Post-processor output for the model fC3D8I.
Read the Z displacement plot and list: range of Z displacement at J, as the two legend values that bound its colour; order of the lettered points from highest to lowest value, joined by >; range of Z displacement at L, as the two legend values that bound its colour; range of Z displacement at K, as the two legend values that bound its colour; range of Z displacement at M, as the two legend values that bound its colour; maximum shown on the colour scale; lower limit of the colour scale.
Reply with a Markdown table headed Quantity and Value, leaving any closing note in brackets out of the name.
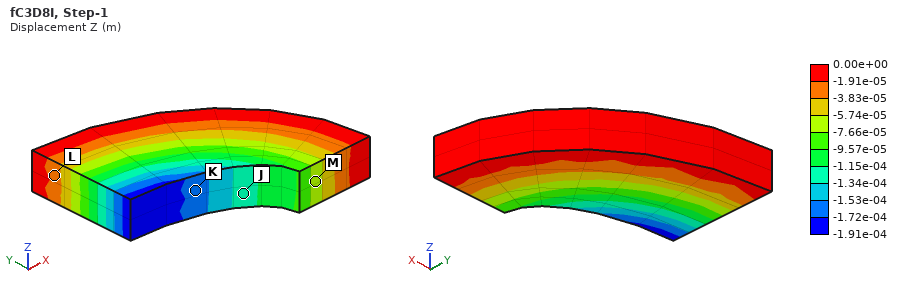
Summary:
| Quantity | Value |
|---|---|
| range of Z displacement at J, as the two legend values that bound its colour | -1.34e-04 to -1.15e-04 m |
| order of the lettered points from highest to lowest value, joined by > | L > M > J > K |
| range of Z displacement at L, as the two legend values that bound its colour | -3.83e-05 to -1.91e-05 m |
| range of Z displacement at K, as the two legend values that bound its colour | -1.72e-04 to -1.53e-04 m |
| range of Z displacement at M, as the two legend values that bound its colour | -7.66e-05 to -5.74e-05 m |
| maximum shown on the colour scale | 0.00e+00 m |
| lower limit of the colour scale | -1.91e-04 m |
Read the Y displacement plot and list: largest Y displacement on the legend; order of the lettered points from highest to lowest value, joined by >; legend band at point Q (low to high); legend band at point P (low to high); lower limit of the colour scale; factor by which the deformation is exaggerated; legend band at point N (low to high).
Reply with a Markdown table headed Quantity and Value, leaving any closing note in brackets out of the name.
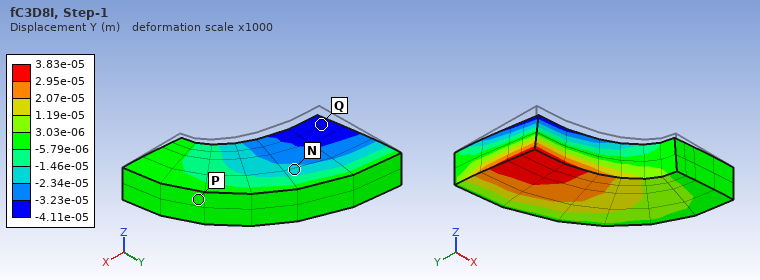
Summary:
| Quantity | Value |
|---|---|
| largest Y displacement on the legend | 3.83e-05 m |
| order of the lettered points from highest to lowest value, joined by > | P > N > Q |
| legend band at point Q | -4.11e-05 to -3.23e-05 m |
| legend band at point P | -5.79e-06 to 3.03e-06 m |
| lower limit of the colour scale | -4.11e-05 m |
| factor by which the deformation is exaggerated | 1000 |
| legend band at point N | -2.34e-05 to -1.46e-05 m |
